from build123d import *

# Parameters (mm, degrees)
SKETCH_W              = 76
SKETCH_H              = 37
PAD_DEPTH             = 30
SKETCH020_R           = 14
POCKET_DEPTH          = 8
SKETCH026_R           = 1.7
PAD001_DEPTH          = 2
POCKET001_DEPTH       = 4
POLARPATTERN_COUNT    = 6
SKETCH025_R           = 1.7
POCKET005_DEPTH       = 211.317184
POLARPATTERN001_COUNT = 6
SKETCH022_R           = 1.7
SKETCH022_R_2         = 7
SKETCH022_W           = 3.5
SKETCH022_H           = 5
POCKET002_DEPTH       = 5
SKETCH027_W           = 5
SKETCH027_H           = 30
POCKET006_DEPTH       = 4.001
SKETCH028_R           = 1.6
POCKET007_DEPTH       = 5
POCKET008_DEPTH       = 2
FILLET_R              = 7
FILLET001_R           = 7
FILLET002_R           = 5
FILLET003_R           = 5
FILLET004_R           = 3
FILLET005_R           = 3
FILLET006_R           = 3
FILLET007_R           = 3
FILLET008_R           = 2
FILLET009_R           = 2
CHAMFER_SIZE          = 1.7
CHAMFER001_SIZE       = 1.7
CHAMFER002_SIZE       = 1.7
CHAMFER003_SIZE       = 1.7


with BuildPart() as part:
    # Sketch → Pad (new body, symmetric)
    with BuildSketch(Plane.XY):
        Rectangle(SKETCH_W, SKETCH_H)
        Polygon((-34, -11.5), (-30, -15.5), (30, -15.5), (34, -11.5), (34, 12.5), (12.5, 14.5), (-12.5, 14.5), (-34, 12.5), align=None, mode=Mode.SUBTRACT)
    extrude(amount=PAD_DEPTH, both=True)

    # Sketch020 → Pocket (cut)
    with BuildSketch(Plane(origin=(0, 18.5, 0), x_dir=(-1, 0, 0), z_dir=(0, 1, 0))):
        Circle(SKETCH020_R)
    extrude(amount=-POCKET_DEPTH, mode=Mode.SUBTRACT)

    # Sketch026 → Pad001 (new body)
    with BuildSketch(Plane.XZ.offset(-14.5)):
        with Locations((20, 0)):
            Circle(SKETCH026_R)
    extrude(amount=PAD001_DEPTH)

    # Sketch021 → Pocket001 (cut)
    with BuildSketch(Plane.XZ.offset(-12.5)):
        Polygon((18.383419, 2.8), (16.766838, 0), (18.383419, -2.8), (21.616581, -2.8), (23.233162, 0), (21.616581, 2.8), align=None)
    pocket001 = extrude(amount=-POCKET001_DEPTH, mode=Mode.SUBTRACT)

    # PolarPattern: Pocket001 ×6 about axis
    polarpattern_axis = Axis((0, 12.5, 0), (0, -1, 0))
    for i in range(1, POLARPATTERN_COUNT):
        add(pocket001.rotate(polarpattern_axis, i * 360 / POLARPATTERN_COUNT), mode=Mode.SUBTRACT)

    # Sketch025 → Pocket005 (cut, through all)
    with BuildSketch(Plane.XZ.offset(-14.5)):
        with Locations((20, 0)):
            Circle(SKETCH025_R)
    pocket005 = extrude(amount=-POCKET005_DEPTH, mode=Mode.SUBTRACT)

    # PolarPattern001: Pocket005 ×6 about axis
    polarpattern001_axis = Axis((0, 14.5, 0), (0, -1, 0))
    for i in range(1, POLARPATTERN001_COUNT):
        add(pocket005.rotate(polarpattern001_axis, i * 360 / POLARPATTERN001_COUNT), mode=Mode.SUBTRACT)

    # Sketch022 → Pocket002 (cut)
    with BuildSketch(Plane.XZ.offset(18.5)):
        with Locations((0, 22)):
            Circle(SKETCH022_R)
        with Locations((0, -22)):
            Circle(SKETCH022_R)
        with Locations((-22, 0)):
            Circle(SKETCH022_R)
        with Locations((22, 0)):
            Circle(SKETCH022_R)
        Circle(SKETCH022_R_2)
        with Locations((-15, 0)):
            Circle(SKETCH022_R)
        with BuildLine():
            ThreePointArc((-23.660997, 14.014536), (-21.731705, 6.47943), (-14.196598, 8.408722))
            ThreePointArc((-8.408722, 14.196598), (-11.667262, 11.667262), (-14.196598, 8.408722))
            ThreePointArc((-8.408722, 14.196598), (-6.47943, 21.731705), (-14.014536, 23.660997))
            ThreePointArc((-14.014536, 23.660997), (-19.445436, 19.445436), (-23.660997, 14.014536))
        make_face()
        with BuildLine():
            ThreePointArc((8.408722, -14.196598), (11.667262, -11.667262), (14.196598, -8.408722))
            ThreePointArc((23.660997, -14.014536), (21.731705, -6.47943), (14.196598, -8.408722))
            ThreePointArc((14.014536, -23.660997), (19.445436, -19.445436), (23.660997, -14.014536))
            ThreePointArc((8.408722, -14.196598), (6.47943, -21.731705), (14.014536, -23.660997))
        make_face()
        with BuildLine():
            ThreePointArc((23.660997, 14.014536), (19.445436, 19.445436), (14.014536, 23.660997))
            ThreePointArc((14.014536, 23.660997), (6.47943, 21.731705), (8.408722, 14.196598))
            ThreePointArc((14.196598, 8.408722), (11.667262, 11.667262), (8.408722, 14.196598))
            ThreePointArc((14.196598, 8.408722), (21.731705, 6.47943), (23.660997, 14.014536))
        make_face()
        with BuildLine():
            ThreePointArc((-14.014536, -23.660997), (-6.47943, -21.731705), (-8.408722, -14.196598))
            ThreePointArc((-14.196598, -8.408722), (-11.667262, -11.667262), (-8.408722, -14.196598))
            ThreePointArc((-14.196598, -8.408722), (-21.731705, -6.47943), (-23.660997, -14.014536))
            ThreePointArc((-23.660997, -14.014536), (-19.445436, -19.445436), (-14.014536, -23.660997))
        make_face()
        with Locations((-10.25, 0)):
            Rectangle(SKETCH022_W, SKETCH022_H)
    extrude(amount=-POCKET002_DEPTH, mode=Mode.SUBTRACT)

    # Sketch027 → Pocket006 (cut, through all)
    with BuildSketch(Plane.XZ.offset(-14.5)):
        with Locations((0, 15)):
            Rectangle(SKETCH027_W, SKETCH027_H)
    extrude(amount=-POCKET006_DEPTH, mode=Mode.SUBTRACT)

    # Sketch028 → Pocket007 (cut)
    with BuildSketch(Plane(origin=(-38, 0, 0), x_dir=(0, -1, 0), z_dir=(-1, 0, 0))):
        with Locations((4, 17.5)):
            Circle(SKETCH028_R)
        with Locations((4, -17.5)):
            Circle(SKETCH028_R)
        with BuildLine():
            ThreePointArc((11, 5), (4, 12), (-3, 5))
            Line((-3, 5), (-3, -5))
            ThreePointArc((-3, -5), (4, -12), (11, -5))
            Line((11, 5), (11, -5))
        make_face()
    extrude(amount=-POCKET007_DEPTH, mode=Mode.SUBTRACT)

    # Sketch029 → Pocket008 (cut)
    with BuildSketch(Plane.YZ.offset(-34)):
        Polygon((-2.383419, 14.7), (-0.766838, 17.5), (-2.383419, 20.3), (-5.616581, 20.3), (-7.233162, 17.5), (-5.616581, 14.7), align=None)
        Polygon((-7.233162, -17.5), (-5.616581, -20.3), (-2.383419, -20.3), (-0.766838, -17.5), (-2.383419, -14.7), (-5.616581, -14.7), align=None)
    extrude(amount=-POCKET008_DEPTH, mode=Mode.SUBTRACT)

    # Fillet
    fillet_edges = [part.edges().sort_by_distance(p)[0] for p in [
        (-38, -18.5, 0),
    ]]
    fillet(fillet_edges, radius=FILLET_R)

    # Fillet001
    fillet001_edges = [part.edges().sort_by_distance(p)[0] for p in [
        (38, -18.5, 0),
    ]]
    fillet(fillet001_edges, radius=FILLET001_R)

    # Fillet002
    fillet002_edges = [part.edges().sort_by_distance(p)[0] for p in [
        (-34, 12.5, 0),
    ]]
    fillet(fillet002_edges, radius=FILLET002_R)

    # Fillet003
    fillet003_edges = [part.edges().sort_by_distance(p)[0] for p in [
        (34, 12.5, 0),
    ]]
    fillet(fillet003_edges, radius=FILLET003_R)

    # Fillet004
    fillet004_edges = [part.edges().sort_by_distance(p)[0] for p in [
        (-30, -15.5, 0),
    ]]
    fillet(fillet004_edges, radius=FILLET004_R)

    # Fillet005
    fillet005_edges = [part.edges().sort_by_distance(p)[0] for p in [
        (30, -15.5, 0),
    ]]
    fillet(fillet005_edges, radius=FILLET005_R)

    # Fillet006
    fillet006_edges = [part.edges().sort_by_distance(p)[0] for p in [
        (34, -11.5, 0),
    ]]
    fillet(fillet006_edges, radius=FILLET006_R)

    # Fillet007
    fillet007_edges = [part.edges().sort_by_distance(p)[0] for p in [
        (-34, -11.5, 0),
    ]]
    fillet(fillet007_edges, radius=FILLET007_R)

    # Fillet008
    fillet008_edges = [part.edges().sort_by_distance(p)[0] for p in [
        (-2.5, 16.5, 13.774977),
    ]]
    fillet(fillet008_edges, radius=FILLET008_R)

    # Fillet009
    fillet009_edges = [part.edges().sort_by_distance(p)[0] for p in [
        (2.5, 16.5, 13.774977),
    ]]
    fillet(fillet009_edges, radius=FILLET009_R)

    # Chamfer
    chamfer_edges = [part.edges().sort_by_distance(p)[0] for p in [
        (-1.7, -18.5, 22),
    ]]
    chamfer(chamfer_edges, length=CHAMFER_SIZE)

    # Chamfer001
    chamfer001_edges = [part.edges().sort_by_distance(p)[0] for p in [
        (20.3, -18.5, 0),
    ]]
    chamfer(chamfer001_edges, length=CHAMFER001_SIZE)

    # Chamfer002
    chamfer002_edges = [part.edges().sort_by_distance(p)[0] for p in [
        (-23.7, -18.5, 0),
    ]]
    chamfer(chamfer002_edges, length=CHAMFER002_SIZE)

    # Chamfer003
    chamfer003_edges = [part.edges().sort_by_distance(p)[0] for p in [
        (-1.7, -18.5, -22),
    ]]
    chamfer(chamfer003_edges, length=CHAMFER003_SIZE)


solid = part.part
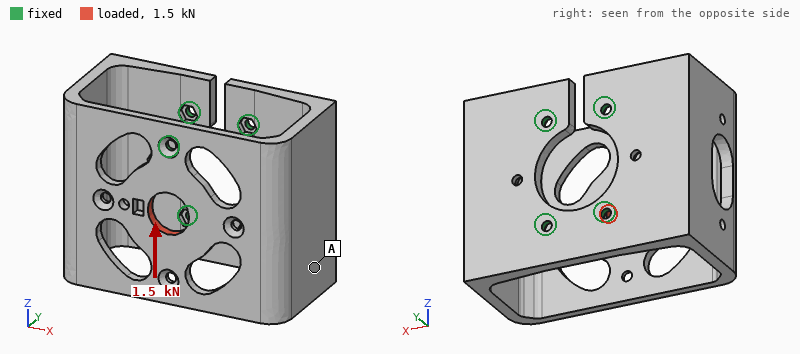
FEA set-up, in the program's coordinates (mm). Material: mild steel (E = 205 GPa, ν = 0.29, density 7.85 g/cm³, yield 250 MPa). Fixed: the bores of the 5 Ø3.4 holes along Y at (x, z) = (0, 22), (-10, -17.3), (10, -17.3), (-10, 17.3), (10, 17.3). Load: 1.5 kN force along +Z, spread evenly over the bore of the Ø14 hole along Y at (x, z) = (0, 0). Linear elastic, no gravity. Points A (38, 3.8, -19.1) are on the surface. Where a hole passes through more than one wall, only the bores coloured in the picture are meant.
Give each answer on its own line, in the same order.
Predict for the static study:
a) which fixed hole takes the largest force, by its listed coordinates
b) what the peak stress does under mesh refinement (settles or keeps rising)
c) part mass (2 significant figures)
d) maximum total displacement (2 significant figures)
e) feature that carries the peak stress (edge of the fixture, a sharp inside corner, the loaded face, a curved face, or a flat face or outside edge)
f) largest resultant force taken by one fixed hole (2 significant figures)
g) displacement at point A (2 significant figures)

(0, 22)
keeps rising
320 g
8.8 µm
edge of the fixture
1.4 kN
2.9 µm
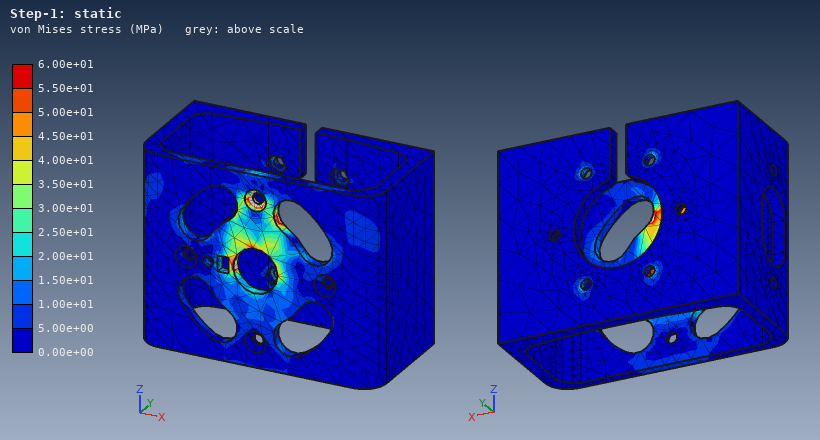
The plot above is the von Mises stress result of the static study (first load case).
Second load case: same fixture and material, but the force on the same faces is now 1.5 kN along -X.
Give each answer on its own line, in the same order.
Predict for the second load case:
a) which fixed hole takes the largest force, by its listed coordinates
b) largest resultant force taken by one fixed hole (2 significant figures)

(0, 22)
1.4 kN
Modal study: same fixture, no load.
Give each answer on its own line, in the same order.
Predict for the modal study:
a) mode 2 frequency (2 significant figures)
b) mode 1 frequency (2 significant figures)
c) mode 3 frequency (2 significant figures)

2100 Hz
2100 Hz
2900 Hz
